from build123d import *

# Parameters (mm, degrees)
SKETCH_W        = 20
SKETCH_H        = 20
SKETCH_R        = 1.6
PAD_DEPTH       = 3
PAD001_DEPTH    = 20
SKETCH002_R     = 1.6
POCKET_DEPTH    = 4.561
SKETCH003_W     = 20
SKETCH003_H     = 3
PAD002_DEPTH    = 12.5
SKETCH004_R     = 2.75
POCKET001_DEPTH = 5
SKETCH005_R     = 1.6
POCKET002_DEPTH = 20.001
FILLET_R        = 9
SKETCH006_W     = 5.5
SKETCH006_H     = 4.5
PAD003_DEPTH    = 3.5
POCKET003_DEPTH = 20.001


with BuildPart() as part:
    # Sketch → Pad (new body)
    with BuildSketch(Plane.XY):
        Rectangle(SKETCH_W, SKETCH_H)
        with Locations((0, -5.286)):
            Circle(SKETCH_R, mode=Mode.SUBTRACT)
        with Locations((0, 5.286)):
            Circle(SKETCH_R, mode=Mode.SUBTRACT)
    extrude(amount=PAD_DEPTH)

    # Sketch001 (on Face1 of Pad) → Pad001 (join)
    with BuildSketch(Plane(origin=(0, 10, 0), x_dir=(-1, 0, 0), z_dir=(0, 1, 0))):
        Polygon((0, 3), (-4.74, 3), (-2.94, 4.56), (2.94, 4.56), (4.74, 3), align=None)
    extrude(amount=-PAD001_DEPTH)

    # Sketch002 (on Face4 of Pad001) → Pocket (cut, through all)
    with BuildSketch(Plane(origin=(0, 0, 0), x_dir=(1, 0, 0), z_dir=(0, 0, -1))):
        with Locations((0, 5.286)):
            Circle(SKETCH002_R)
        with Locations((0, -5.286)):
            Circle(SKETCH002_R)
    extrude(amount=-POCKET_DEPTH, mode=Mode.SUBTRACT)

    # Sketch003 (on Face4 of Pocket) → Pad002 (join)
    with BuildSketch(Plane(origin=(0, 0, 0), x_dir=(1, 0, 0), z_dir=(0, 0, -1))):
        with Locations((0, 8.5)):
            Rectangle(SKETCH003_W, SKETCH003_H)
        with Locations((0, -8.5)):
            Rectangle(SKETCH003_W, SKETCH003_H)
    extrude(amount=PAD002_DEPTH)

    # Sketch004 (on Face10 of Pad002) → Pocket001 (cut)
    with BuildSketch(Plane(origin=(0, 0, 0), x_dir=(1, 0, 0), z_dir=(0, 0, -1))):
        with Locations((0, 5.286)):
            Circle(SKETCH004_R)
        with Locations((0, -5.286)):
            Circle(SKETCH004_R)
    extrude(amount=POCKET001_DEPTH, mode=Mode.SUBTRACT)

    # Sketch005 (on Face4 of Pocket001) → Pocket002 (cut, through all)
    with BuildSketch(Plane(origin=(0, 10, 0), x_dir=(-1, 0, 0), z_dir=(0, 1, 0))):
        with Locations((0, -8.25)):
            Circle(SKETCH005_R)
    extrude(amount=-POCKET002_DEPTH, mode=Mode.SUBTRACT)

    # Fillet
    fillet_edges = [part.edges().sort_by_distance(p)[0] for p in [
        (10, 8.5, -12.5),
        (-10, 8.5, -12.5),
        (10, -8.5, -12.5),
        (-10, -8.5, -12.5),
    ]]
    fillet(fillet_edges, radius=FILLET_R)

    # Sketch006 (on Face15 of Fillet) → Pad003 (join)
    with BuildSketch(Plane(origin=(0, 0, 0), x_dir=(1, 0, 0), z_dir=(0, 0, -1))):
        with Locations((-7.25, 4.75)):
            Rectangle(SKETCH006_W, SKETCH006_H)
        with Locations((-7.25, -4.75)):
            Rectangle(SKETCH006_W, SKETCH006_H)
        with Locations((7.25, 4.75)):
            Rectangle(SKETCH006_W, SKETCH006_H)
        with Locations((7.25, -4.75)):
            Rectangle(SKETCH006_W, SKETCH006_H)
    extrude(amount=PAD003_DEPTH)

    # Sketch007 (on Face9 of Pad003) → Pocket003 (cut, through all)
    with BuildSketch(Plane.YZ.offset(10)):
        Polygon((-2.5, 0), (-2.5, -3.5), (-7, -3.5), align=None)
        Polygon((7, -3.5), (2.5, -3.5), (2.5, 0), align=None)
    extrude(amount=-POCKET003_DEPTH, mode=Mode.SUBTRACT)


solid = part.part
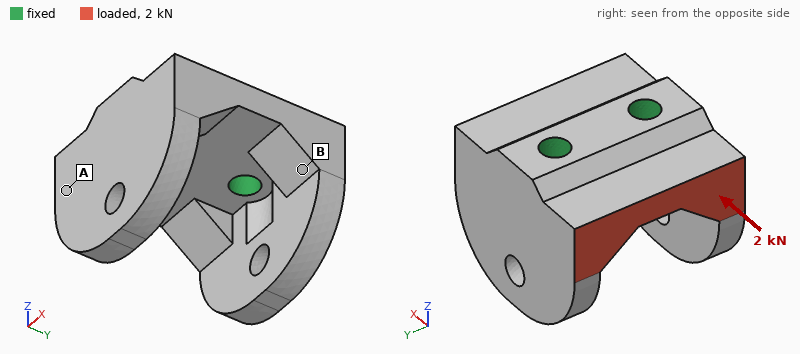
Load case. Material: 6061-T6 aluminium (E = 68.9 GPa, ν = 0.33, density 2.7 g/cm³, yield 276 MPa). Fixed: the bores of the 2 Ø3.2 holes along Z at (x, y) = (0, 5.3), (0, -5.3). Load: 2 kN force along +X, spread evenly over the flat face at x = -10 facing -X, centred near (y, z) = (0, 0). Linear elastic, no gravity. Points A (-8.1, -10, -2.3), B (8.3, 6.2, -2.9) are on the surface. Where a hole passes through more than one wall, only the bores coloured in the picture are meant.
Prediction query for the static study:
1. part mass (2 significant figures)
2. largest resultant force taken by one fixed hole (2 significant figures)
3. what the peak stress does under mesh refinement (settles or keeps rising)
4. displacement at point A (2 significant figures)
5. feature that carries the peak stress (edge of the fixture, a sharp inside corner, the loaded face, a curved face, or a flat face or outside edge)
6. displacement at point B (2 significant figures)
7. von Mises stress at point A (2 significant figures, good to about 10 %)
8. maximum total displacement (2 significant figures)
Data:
7.4 g
1.0 kN
keeps rising
8.0 µm
edge of the fixture
6.1 µm
17 MPa
11 µm
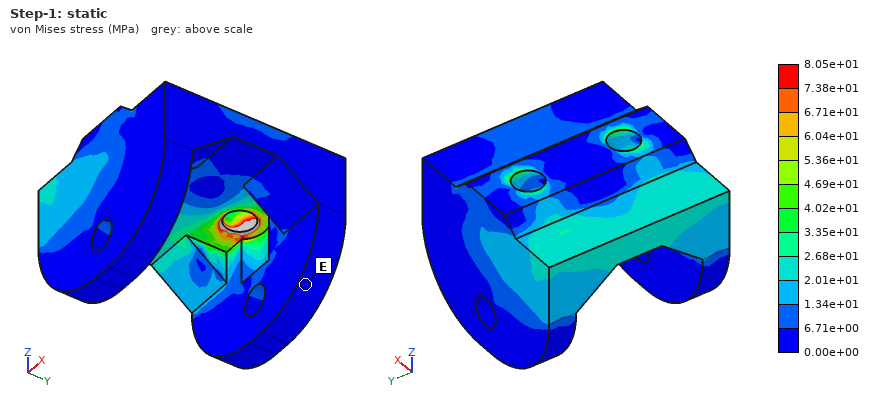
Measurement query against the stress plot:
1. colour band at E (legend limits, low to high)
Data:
0.00e+00 to 6.71e+00 MPa
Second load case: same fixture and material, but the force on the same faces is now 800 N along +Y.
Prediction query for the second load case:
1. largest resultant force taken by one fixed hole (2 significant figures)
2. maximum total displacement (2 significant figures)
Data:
700 N
9.5 µm
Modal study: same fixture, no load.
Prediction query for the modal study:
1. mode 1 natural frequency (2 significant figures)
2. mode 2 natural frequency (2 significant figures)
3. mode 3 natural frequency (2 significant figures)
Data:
16 kHz
17 kHz
17 kHz
